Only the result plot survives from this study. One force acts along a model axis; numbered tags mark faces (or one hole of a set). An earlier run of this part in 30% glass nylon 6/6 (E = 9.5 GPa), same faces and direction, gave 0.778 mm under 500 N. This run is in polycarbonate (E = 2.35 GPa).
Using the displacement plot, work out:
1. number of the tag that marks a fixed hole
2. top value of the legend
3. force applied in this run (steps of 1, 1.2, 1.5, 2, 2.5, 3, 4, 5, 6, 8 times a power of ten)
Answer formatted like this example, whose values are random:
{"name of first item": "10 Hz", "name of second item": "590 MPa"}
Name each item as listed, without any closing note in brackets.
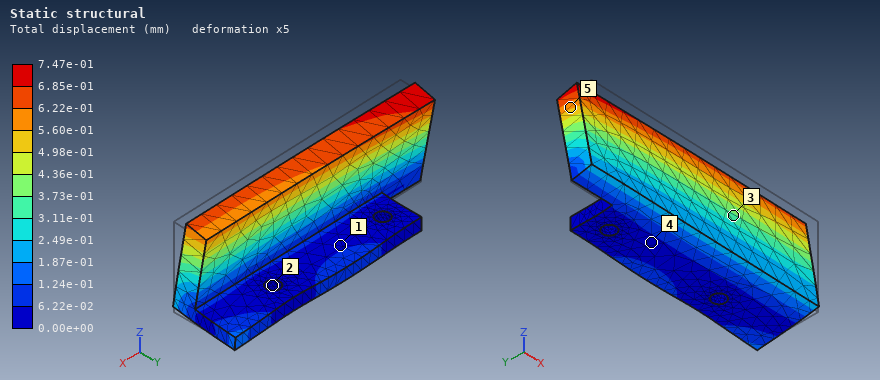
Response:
{"number of the tag that marks a fixed hole": "2", "top value of the legend": "7.47e-01 mm", "force applied in this run": "120 N"}
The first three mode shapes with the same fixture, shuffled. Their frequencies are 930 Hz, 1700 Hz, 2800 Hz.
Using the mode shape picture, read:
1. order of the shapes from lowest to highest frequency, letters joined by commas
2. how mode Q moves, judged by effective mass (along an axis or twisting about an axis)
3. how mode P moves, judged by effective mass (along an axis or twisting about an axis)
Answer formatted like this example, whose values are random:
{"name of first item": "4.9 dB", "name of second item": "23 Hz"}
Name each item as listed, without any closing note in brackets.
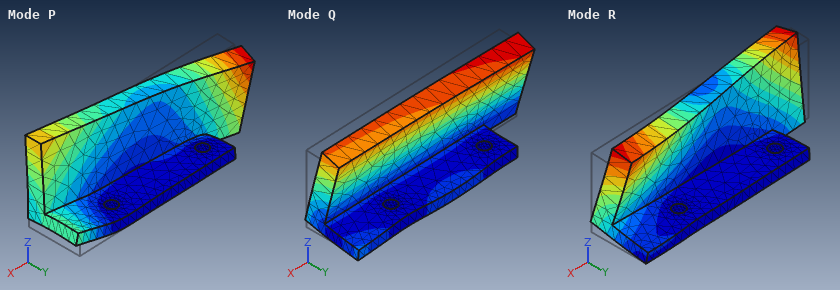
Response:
{"order of the shapes from lowest to highest frequency, letters joined by commas": "Q, R, P", "how mode Q moves, judged by effective mass": "along Y", "how mode P moves, judged by effective mass": "along X"}
